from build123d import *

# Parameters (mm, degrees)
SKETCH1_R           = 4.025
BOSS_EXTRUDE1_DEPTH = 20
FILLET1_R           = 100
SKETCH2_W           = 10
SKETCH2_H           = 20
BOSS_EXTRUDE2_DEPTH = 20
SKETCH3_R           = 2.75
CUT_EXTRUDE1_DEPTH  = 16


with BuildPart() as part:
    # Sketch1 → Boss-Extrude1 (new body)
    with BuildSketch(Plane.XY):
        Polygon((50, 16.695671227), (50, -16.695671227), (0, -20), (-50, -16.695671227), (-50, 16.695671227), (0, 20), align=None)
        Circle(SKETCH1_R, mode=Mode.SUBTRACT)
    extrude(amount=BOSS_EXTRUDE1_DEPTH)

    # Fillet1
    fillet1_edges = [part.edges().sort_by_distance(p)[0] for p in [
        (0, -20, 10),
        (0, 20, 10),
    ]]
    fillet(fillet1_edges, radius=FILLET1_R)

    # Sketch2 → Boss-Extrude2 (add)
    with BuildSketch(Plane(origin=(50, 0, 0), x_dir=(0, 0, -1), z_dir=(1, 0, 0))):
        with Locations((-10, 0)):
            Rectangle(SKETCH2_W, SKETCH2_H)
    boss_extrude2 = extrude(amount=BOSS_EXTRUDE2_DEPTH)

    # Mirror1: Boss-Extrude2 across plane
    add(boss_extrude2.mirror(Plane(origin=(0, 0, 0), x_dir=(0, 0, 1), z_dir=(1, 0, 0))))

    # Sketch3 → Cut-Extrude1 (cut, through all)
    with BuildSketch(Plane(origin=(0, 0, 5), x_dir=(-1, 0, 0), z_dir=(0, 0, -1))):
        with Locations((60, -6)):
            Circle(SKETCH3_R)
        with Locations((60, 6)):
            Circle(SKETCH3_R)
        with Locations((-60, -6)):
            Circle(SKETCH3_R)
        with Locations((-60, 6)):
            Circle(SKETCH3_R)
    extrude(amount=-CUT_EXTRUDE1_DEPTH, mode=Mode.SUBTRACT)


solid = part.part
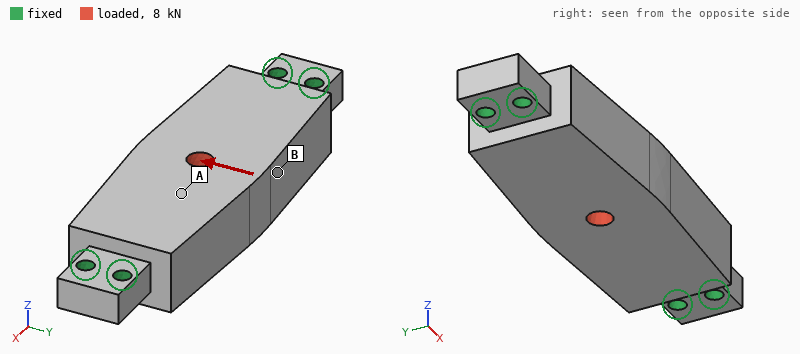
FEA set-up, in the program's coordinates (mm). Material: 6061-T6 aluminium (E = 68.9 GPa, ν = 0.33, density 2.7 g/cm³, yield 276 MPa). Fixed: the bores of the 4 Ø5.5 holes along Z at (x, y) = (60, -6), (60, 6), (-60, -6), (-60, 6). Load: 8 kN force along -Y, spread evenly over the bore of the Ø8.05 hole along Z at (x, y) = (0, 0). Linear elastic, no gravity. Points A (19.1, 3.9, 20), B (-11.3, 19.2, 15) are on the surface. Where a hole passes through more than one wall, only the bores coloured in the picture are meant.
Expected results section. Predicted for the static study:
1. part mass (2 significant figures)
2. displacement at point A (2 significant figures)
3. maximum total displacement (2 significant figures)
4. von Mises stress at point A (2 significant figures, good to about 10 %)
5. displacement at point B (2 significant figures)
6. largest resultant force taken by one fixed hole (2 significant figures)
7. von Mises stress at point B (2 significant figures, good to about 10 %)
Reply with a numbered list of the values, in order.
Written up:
1. 210 g
2. 38 µm
3. 47 µm
4. 12 MPa
5. 41 µm
6. 3.8 kN
7. 31 MPa
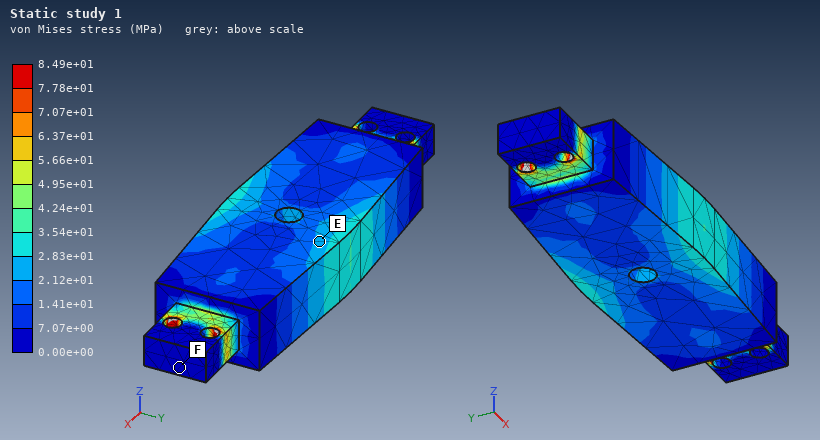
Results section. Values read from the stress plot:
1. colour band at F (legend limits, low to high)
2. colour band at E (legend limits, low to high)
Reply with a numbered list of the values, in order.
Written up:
1. 0.00e+00 to 7.07e+00 MPa
2. 2.12e+01 to 2.83e+01 MPa
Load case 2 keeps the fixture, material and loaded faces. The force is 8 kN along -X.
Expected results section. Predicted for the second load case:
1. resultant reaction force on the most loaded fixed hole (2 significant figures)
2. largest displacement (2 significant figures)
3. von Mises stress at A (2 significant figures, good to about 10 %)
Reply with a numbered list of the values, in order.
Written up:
1. 2.0 kN
2. 8.6 µm
3. 8.1 MPa
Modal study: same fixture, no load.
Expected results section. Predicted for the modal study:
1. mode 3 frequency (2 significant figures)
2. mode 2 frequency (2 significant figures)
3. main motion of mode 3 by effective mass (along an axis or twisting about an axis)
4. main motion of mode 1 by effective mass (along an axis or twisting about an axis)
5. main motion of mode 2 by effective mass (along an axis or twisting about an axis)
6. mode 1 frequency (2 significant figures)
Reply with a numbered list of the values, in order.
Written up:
1. 6200 Hz
2. 5000 Hz
3. along Y
4. along Z
5. twisting about X
6. 3900 Hz
